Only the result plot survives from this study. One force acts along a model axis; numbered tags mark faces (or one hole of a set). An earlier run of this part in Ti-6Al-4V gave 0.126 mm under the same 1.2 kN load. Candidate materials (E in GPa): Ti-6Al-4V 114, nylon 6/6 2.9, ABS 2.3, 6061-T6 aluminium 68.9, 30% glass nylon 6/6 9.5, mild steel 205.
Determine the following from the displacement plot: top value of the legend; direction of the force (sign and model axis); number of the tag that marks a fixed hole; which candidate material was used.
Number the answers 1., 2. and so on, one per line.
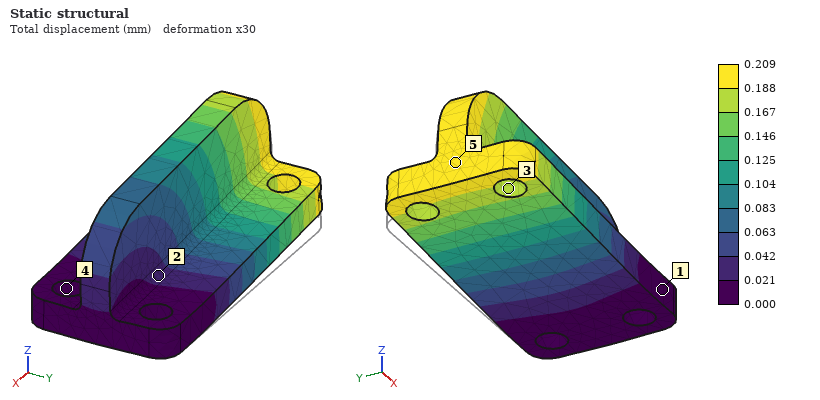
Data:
1. 0.209 mm
2. +Z
3. 4
4. 6061-T6 aluminium
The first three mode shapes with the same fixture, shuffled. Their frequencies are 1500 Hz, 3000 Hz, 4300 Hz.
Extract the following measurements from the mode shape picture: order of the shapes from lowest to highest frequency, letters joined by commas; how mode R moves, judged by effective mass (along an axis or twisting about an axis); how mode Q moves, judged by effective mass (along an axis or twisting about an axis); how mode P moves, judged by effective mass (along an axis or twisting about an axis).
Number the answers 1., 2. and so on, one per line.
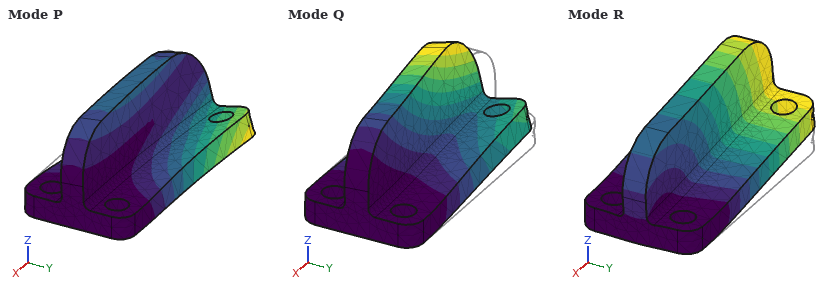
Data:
1. R, Q, P
2. along Z
3. along Y
4. along Y
